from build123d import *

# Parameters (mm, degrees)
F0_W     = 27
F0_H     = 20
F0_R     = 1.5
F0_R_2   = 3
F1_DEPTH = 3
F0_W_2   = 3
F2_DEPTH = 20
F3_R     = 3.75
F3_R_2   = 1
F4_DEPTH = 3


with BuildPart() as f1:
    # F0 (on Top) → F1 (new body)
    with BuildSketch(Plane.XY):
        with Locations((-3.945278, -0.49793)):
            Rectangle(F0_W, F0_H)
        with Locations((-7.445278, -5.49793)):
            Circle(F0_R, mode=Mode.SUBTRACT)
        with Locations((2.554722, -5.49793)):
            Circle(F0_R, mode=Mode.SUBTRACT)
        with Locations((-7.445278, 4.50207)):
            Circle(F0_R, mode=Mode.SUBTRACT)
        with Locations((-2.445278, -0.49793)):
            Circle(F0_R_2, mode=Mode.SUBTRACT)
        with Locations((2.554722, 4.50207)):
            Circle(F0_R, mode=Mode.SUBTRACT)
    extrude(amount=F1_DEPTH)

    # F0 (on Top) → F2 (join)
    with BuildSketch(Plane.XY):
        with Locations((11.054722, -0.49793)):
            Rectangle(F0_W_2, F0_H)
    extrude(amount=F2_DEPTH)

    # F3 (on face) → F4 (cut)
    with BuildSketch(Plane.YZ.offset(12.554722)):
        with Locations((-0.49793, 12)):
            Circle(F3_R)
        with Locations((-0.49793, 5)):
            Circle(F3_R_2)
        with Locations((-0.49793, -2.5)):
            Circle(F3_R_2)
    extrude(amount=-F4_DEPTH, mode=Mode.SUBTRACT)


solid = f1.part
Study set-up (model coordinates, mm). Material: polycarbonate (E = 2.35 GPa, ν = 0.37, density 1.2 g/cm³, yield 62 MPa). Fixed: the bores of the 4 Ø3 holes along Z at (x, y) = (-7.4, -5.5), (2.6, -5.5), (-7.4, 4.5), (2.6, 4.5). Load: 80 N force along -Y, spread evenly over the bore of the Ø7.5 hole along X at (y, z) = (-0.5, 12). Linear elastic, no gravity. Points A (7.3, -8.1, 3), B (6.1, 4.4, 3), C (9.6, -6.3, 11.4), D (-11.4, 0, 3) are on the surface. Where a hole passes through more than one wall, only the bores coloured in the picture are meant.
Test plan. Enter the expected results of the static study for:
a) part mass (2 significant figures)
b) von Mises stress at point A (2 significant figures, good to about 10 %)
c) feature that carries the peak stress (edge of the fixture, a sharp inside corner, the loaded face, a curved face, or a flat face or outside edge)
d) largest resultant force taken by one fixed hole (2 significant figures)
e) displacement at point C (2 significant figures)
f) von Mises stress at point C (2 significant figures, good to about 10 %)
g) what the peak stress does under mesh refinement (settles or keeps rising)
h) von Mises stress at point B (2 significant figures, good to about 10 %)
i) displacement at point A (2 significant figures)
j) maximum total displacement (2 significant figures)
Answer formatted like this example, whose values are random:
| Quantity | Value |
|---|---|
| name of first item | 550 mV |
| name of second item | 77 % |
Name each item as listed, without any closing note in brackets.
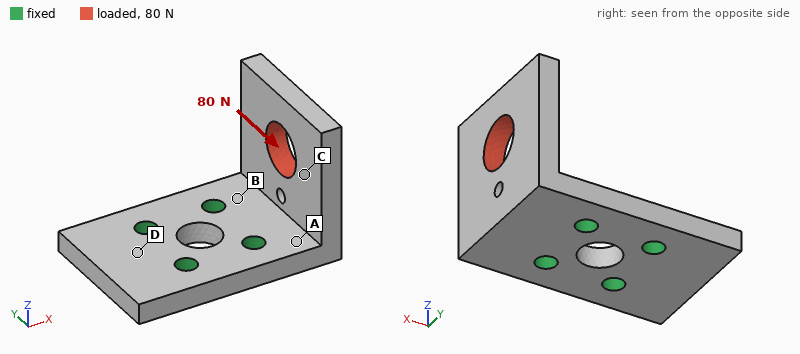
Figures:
| Quantity | Value |
|---|---|
| part mass | 3.0 g |
| von Mises stress at point A | 11 MPa |
| feature that carries the peak stress | edge of the fixture |
| largest resultant force taken by one fixed hole | 89 N |
| displacement at point C | 0.24 mm |
| von Mises stress at point C | 5.6 MPa |
| what the peak stress does under mesh refinement | keeps rising |
| von Mises stress at point B | 13 MPa |
| displacement at point A | 0.071 mm |
| maximum total displacement | 0.44 mm |
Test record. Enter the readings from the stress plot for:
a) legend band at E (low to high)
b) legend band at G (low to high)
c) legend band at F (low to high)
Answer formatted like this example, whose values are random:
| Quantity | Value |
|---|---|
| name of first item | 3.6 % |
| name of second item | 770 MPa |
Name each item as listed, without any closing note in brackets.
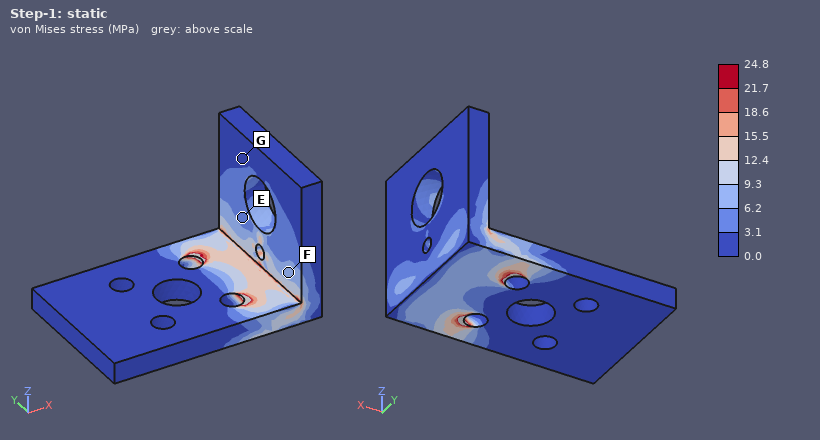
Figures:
| Quantity | Value |
|---|---|
| legend band at E | 3.1 to 6.2 MPa |
| legend band at G | 0.0 to 3.1 MPa |
| legend band at F | 6.2 to 9.3 MPa |
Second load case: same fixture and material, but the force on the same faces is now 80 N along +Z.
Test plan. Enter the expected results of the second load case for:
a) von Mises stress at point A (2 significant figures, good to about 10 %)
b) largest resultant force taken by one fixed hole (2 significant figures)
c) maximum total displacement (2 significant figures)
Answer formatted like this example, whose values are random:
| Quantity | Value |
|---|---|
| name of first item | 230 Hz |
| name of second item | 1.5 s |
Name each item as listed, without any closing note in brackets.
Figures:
| Quantity | Value |
|---|---|
| von Mises stress at point A | 8.9 MPa |
| largest resultant force taken by one fixed hole | 44 N |
| maximum total displacement | 0.47 mm |
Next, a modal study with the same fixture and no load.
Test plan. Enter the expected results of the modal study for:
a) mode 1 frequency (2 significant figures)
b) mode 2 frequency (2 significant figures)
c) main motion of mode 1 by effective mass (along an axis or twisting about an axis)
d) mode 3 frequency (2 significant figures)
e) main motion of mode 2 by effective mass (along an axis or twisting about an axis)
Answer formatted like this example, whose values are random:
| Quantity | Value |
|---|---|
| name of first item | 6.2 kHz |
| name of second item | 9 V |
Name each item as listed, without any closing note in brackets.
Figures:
| Quantity | Value |
|---|---|
| mode 1 frequency | 1300 Hz |
| mode 2 frequency | 2400 Hz |
| main motion of mode 1 by effective mass | along X |
| mode 3 frequency | 3700 Hz |
| main motion of mode 2 by effective mass | along Y |
